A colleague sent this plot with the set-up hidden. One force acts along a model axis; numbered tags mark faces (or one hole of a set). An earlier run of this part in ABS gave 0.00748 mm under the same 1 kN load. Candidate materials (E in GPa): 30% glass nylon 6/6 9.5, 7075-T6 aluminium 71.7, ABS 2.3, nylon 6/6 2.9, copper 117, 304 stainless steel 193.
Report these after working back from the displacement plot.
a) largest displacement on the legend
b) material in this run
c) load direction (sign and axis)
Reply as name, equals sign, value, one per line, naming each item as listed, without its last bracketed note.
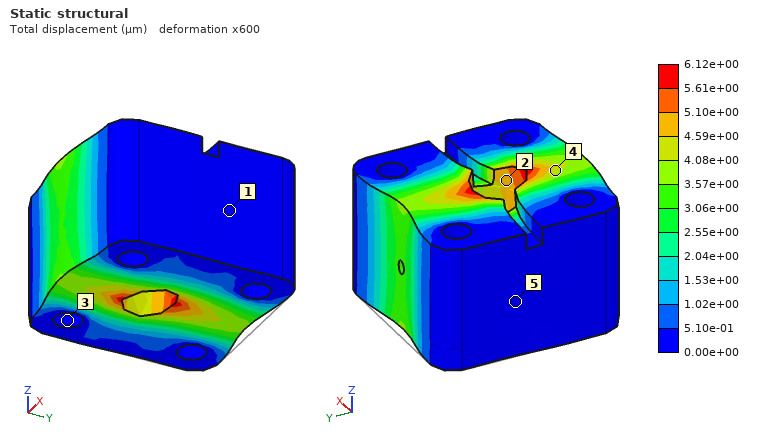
largest displacement on the legend = 6.12e+00 µm
material in this run = nylon 6/6
load direction = -Y
